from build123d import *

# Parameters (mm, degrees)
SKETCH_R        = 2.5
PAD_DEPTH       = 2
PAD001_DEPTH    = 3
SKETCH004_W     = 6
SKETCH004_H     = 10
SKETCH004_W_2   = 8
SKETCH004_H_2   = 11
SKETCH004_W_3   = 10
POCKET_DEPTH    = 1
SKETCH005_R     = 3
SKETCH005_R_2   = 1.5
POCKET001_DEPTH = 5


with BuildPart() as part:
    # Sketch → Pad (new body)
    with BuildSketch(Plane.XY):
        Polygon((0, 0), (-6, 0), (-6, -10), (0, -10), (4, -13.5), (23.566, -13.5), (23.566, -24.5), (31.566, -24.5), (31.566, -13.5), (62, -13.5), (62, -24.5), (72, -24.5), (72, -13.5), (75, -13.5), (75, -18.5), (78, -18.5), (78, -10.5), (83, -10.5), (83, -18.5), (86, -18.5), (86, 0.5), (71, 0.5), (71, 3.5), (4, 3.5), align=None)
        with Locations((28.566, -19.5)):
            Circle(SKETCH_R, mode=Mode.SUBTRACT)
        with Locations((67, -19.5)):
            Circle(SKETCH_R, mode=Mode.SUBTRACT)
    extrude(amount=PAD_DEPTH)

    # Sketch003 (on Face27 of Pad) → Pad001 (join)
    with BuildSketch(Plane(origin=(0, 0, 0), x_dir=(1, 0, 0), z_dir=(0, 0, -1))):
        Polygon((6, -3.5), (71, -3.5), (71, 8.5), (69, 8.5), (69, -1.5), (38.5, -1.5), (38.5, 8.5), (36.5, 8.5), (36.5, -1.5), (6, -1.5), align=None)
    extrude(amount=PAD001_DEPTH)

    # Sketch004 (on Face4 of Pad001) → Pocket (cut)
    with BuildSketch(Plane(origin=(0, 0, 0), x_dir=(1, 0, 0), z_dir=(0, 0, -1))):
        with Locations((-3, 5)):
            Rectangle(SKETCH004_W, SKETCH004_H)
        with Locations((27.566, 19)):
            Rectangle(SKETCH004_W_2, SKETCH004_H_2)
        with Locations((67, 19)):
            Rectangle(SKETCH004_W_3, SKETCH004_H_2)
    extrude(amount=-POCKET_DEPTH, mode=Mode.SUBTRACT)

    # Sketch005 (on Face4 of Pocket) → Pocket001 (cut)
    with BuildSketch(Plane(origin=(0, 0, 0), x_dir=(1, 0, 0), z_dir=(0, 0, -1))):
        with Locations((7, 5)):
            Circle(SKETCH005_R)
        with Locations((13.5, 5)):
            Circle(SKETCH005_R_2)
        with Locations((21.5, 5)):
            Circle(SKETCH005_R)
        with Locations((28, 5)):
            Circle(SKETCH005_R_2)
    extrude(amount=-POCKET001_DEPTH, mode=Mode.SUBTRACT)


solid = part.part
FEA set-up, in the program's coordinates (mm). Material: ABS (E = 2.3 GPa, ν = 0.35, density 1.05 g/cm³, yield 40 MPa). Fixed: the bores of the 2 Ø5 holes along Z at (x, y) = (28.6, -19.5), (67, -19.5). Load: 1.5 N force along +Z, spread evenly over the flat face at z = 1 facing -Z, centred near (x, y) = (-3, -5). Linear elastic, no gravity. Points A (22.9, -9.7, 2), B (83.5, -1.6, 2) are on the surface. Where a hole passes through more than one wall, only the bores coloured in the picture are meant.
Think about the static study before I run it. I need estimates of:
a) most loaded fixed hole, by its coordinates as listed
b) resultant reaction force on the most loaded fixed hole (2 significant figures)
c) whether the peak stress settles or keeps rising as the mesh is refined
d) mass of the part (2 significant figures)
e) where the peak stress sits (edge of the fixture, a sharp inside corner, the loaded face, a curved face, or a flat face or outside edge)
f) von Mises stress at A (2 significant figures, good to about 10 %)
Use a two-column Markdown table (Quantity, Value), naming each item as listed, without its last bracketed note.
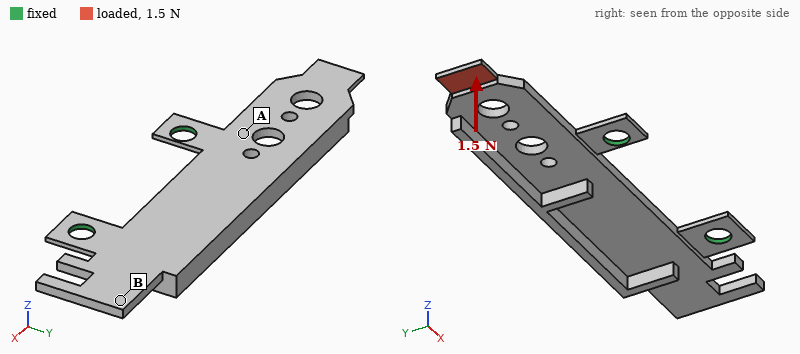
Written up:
| Quantity | Value |
|---|---|
| most loaded fixed hole, by its coordinates as listed | (28.6, -19.5) |
| resultant reaction force on the most loaded fixed hole | 2.5 N |
| whether the peak stress settles or keeps rising as the mesh is refined | keeps rising |
| mass of the part | 3.6 g |
| where the peak stress sits | edge of the fixture |
| von Mises stress at A | 2.5 MPa |
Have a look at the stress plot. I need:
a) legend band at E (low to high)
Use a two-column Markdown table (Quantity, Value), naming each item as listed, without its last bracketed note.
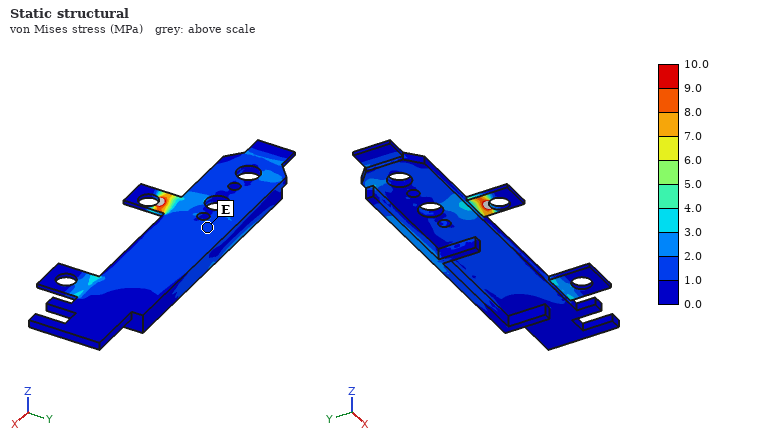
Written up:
| Quantity | Value |
|---|---|
| legend band at E | 1.0 to 2.0 MPa |
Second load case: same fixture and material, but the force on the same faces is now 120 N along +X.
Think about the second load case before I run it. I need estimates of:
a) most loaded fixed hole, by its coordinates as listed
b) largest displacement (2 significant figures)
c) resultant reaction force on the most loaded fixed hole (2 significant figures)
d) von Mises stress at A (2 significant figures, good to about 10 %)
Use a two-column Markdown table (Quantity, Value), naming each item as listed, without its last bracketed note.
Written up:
| Quantity | Value |
|---|---|
| most loaded fixed hole, by its coordinates as listed | (28.6, -19.5) |
| largest displacement | 0.42 mm |
| resultant reaction force on the most loaded fixed hole | 72 N |
| von Mises stress at A | 5.9 MPa |
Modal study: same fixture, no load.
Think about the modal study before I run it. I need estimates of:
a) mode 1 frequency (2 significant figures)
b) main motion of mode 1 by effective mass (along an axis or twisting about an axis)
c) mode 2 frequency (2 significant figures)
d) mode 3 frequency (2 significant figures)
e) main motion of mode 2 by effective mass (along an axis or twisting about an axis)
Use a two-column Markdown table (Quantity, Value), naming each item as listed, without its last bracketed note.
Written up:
| Quantity | Value |
|---|---|
| mode 1 frequency | 200 Hz |
| main motion of mode 1 by effective mass | along Z |
| mode 2 frequency | 400 Hz |
| mode 3 frequency | 770 Hz |
| main motion of mode 2 by effective mass | twisting about Y |
